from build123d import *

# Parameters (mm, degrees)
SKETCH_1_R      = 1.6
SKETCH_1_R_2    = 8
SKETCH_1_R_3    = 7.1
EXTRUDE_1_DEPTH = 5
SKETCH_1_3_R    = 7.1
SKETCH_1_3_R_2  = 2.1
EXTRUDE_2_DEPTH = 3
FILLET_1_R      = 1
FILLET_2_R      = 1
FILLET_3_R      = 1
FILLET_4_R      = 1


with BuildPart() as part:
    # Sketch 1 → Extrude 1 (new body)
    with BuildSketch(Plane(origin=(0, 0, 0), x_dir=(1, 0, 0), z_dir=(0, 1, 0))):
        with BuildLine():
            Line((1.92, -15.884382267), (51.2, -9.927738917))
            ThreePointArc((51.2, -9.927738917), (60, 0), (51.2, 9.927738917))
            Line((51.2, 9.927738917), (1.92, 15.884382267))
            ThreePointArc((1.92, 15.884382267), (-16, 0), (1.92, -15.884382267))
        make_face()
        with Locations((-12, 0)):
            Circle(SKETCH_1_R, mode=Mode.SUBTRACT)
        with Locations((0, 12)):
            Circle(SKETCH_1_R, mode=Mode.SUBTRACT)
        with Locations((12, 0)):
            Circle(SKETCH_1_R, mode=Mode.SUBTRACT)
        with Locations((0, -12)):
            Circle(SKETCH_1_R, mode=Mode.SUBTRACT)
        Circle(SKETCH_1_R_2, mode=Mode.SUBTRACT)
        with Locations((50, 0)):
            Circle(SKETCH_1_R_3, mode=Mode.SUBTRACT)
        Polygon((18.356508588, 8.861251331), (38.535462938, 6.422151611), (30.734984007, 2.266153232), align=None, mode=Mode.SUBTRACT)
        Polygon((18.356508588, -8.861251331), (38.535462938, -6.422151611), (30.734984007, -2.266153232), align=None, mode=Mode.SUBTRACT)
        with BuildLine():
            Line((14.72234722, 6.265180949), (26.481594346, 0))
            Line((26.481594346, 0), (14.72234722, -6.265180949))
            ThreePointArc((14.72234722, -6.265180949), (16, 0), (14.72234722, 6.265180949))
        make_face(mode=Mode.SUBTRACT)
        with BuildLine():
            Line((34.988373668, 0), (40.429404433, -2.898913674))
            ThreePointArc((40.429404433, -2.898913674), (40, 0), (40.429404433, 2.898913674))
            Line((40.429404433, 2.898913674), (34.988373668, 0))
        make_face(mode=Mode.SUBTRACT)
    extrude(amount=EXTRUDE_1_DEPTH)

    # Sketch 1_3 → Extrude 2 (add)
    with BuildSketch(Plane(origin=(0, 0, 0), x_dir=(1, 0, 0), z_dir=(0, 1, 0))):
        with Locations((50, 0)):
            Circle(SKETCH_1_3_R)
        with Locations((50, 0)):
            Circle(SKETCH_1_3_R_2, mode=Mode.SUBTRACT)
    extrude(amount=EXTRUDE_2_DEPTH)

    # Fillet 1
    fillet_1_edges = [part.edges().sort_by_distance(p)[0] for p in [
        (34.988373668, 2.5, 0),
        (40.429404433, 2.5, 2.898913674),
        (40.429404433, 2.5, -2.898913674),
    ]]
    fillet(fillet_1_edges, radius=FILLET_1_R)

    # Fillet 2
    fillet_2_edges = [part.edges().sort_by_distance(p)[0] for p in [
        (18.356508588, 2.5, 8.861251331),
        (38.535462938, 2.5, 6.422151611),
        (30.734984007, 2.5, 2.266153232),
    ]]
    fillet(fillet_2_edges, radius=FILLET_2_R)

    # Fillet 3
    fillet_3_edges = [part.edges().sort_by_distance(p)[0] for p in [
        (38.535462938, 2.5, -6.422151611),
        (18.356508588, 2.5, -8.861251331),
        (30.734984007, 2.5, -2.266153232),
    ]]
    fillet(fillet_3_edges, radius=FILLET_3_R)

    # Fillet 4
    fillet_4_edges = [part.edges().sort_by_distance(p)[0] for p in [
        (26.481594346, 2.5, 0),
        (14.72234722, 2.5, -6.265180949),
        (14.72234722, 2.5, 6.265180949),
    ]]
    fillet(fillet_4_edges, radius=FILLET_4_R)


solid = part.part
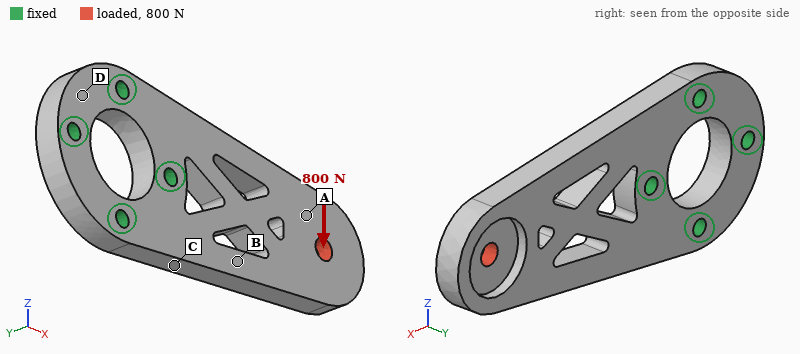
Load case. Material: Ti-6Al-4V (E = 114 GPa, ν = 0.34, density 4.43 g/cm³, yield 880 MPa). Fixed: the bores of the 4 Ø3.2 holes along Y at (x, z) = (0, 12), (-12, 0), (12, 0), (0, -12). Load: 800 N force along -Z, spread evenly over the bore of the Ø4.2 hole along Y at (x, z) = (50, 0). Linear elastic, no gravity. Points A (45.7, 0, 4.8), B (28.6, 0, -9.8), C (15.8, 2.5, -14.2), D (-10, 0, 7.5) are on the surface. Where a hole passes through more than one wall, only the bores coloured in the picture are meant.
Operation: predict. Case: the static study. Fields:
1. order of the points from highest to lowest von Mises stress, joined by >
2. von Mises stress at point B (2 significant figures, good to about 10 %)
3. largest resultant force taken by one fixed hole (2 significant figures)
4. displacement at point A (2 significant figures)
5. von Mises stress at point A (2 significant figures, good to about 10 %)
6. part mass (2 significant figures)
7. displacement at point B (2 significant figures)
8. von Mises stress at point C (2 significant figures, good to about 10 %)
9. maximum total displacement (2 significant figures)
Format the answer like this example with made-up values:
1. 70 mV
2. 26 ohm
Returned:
1. C > B > A > D
2. 35 MPa
3. 1.2 kN
4. 38 µm
5. 22 MPa
6. 31 g
7. 18 µm
8. 53 MPa
9. 54 µm
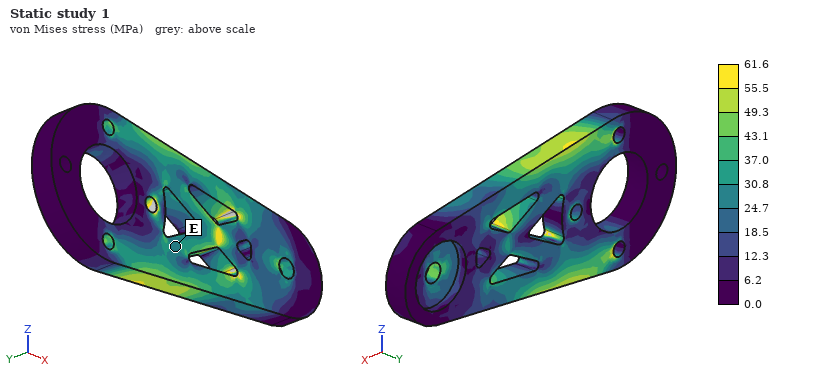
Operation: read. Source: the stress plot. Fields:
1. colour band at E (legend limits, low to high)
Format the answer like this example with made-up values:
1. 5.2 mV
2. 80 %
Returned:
1. 24.7 to 30.8 MPa
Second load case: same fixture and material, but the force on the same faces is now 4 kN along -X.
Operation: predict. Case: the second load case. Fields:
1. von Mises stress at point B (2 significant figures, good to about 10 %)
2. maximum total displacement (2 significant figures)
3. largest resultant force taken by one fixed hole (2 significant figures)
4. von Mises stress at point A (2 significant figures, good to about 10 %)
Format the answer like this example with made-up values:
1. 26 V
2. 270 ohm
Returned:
1. 110 MPa
2. 0.23 mm
3. 1.5 kN
4. 79 MPa
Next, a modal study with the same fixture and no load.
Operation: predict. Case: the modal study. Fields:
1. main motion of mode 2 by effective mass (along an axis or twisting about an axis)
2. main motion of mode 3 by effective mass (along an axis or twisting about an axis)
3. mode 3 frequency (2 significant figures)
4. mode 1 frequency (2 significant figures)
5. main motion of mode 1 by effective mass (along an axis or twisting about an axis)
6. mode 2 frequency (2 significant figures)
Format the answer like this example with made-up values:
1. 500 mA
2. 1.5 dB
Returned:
1. twisting about X
2. along Z
3. 7700 Hz
4. 1800 Hz
5. along Y
6. 6400 Hz
